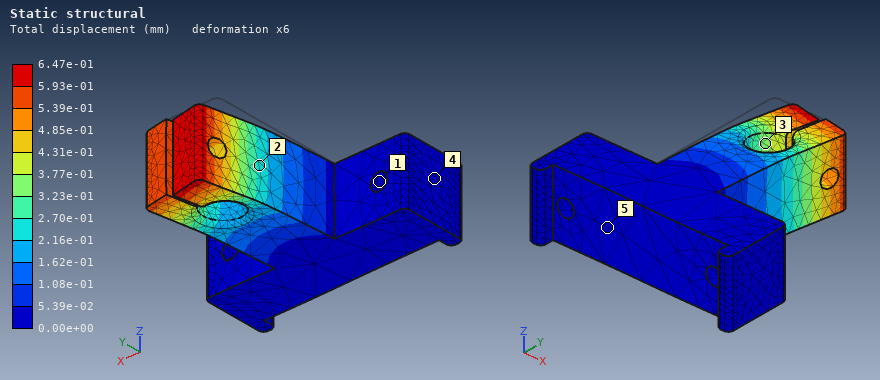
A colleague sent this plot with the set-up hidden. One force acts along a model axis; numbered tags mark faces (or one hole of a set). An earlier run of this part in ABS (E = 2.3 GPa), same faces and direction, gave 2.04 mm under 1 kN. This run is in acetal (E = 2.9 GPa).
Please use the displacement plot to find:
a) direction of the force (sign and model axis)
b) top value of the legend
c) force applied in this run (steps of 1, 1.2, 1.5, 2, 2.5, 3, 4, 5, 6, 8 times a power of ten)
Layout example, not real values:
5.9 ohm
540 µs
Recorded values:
+X
6.47e-01 mm
400 N
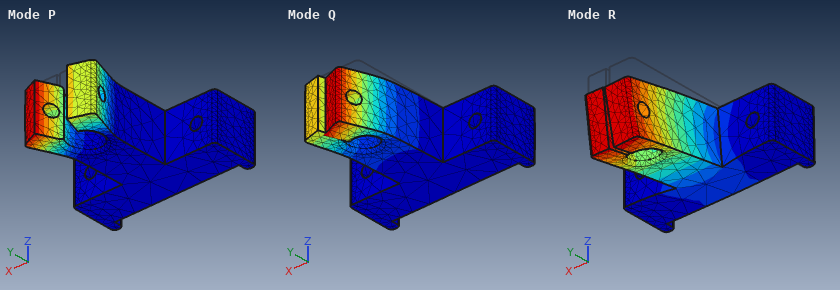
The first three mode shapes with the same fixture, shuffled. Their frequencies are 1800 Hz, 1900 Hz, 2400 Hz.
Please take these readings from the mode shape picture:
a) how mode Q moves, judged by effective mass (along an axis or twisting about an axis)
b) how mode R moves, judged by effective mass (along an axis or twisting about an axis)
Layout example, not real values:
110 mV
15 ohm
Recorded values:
along X
along Z
